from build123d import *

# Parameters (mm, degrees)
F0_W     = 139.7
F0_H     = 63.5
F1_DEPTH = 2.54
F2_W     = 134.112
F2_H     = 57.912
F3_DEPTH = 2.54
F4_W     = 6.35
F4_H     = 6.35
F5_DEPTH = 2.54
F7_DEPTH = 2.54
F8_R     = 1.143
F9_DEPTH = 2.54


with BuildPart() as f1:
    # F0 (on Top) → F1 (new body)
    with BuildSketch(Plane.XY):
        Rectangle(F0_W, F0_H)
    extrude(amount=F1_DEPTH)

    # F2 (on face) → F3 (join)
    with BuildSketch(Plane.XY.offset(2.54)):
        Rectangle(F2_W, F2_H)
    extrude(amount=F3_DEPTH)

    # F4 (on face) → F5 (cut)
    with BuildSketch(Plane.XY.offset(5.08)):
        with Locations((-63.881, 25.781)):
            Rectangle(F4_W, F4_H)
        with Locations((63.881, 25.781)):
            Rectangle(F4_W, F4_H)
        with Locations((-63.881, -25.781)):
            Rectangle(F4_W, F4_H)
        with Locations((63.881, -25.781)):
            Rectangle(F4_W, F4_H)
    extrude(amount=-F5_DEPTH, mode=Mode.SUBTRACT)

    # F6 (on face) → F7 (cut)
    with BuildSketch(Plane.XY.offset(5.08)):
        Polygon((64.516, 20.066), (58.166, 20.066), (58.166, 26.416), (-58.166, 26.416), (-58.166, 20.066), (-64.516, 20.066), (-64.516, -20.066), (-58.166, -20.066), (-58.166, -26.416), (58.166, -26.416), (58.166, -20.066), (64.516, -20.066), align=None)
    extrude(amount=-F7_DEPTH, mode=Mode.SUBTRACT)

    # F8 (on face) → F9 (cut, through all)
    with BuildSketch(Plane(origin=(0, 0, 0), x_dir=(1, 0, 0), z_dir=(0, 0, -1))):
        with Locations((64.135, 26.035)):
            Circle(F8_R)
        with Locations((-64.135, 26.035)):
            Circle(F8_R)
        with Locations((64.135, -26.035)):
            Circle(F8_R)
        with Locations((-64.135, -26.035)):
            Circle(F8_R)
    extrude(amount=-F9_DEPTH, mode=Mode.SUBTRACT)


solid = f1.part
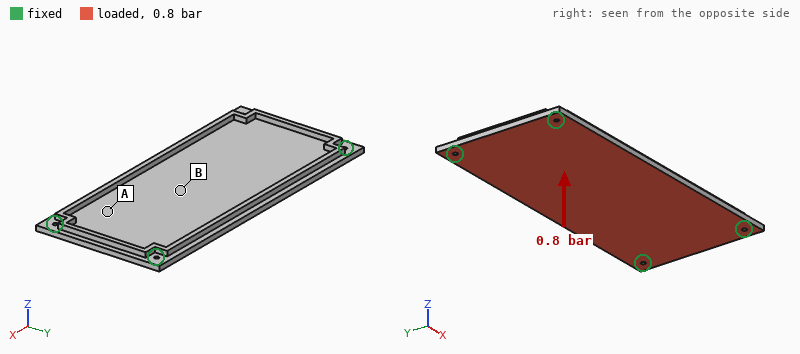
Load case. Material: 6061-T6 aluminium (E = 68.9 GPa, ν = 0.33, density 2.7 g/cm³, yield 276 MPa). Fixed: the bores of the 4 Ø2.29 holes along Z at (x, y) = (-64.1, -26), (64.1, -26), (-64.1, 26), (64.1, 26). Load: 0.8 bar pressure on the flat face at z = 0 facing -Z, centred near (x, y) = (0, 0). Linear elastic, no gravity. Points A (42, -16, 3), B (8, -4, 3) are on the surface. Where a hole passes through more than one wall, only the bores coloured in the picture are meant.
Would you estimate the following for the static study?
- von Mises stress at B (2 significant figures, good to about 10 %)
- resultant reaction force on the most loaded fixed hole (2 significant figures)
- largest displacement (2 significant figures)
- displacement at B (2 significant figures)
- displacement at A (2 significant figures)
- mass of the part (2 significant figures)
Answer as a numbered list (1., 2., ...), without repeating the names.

1. 30 MPa
2. 190 N
3. 0.50 mm
4. 0.49 mm
5. 0.21 mm
6. 67 g
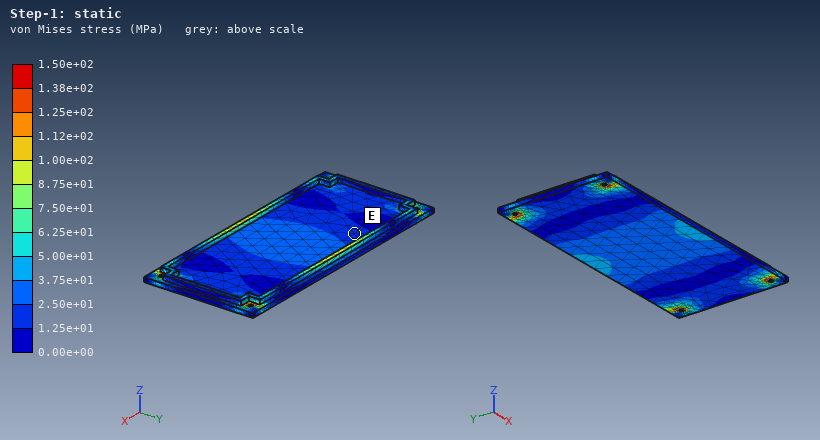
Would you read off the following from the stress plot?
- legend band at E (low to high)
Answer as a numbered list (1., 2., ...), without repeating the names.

1. 1.25e+01 to 2.50e+01 MPa
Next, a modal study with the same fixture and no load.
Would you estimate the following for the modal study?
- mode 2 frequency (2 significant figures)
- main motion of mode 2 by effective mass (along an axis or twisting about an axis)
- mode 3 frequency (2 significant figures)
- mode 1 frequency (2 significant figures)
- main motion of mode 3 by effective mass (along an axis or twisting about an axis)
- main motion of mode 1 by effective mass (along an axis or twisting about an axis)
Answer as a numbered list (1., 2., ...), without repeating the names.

1. 1500 Hz
2. twisting about X
3. 2400 Hz
4. 850 Hz
5. twisting about Y
6. along Z
